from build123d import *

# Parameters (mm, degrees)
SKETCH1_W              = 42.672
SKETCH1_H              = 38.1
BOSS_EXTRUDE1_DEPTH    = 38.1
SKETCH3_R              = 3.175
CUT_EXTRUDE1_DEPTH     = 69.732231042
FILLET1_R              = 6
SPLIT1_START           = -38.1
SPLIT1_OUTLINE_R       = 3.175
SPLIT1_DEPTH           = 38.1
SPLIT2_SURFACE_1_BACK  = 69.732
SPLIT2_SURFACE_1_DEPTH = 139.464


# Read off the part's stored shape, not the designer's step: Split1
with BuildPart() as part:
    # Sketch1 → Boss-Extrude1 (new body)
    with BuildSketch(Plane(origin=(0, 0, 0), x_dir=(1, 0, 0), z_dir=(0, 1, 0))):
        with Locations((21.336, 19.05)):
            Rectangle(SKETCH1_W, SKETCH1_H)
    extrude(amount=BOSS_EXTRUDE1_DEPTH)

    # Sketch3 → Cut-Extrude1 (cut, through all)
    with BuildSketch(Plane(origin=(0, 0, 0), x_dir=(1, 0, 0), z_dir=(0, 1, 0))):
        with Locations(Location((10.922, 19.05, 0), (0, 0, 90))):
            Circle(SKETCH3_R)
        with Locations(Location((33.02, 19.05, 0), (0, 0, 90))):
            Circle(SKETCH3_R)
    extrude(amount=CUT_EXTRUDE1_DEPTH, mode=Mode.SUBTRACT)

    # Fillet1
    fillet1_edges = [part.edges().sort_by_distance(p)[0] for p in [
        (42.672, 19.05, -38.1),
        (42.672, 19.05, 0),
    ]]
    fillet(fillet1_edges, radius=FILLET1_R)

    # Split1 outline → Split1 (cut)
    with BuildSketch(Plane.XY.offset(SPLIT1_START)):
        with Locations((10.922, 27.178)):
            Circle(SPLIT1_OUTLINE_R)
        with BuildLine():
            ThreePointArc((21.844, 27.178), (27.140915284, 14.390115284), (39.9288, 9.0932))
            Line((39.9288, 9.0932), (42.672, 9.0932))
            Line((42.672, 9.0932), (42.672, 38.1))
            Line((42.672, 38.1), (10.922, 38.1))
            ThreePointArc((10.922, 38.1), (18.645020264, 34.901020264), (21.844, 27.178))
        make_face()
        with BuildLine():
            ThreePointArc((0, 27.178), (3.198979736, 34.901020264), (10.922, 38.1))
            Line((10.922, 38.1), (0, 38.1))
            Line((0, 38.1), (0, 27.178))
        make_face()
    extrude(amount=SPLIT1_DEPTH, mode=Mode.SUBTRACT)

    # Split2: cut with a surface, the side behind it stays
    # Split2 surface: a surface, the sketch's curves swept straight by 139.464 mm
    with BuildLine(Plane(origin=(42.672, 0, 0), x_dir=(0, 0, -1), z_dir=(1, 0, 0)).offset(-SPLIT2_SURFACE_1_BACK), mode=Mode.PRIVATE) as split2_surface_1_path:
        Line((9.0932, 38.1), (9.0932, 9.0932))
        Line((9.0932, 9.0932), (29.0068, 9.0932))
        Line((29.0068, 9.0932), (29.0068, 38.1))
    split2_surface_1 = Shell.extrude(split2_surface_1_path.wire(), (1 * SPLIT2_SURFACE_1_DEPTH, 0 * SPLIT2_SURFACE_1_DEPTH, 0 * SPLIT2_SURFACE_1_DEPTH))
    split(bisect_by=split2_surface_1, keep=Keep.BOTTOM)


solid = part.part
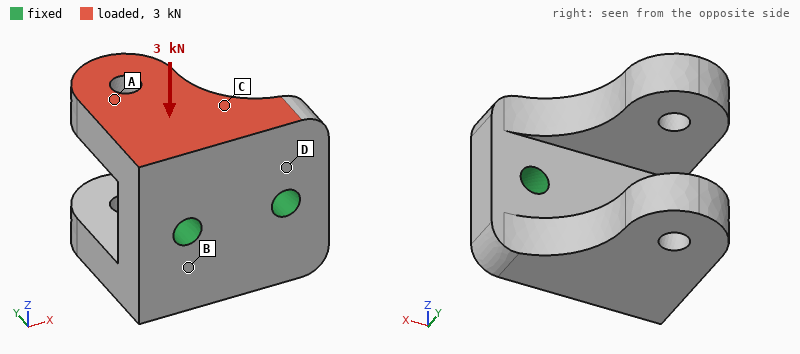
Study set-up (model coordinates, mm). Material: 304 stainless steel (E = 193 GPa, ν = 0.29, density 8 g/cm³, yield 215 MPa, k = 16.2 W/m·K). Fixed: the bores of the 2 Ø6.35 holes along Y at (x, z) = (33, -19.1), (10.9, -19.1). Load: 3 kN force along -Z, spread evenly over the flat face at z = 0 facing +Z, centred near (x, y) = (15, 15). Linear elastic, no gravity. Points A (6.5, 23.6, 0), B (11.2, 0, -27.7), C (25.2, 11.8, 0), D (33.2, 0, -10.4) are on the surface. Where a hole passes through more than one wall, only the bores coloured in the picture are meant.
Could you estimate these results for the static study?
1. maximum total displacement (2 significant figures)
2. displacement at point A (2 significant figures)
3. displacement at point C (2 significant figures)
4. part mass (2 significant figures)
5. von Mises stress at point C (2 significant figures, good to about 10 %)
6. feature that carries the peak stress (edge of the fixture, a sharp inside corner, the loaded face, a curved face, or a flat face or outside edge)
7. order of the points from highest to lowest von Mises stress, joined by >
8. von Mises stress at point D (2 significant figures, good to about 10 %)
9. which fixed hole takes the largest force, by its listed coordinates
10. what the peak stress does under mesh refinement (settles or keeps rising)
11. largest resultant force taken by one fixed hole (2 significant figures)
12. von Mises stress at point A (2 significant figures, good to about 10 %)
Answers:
57 µm
32 µm
13 µm
200 g
55 MPa
edge of the fixture
C > D > A > B
37 MPa
(10.9, -19.1)
keeps rising
2.4 kN
22 MPa
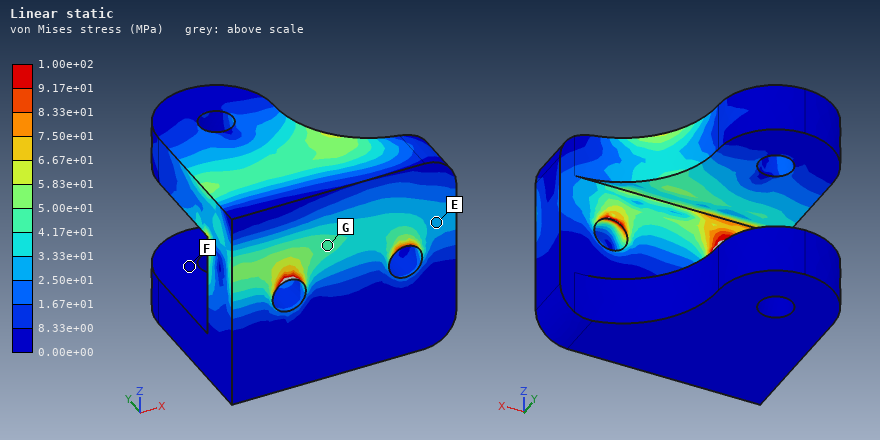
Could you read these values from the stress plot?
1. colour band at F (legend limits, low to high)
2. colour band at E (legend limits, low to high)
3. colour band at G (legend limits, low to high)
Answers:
0.00e+00 to 8.33e+00 MPa
2.50e+01 to 3.33e+01 MPa
4.17e+01 to 5.00e+01 MPa
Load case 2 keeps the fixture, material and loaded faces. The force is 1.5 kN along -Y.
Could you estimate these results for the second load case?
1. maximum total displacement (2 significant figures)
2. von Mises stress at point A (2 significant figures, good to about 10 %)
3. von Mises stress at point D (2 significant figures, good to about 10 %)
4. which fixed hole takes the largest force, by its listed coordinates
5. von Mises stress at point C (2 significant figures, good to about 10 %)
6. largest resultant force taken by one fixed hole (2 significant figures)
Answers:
25 µm
9.7 MPa
25 MPa
(10.9, -19.1)
16 MPa
1.1 kN
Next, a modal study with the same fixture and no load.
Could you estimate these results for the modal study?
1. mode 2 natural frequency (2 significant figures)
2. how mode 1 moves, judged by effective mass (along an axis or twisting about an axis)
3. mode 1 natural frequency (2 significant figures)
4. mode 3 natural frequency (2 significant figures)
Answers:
5600 Hz
along Z
5300 Hz
9700 Hz
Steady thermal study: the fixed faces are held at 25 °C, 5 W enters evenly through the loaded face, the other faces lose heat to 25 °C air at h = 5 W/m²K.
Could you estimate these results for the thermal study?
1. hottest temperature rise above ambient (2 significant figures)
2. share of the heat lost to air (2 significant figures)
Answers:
25 K
4.2 %
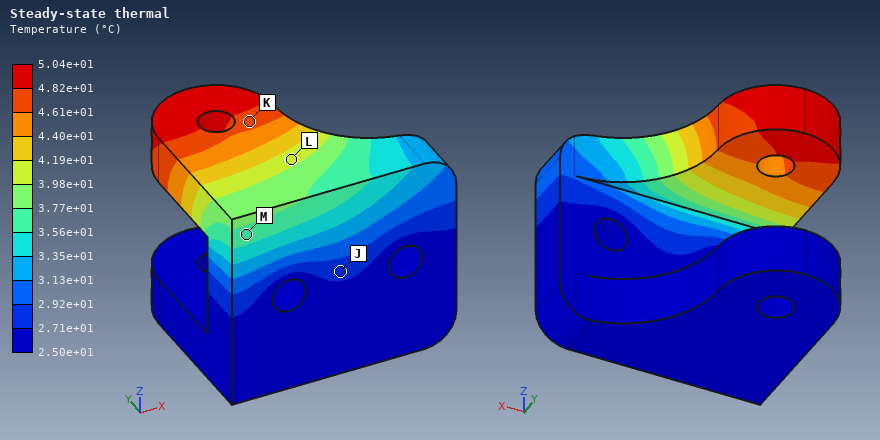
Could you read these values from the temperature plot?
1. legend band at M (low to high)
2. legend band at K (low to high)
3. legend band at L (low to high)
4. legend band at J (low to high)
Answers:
3.56e+01 to 3.77e+01 °C
4.61e+01 to 4.82e+01 °C
3.98e+01 to 4.19e+01 °C
2.71e+01 to 2.92e+01 °C
